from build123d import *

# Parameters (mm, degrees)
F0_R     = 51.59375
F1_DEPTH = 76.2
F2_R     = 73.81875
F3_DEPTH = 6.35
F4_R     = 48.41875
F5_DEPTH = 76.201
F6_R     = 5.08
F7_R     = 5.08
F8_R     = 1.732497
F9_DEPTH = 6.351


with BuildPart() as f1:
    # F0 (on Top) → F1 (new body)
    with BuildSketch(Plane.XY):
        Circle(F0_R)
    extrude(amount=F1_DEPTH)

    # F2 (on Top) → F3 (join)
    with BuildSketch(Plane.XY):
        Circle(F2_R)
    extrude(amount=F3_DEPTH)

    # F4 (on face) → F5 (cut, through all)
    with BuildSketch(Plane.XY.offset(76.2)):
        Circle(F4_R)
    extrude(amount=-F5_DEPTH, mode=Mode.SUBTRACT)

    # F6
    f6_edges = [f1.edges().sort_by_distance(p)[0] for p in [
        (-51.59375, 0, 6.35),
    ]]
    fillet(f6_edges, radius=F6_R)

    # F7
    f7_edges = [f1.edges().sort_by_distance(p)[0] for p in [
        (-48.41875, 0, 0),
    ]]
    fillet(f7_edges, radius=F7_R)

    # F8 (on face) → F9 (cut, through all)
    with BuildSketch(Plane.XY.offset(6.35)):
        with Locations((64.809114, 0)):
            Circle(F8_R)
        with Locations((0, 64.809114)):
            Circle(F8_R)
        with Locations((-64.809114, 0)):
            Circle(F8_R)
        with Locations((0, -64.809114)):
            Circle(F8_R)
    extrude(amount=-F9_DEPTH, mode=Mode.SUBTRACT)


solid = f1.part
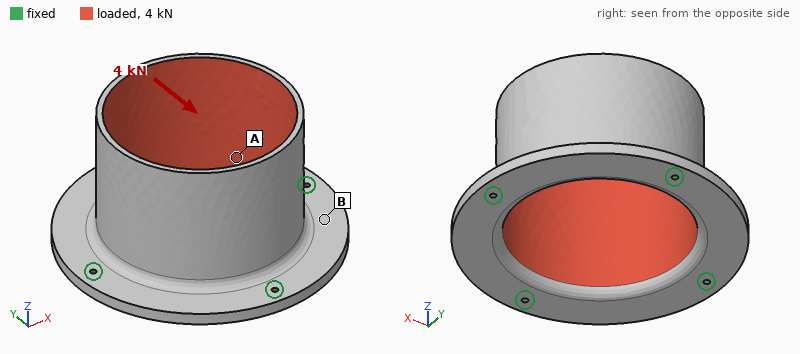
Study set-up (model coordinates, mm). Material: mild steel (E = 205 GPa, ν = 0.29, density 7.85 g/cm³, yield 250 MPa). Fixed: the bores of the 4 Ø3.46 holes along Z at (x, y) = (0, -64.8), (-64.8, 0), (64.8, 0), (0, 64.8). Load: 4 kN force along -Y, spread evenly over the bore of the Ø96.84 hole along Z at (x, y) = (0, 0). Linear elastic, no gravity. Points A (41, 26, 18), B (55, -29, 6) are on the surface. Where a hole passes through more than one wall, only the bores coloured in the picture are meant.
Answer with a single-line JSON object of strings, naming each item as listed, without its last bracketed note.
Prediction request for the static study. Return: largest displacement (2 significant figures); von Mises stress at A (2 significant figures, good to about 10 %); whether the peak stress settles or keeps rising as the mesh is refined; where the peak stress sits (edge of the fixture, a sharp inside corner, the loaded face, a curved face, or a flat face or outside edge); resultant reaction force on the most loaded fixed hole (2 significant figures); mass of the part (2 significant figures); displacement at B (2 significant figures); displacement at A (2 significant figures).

{"largest displacement": "22 µm", "von Mises stress at A": "9.3 MPa", "whether the peak stress settles or keeps rising as the mesh is refined": "keeps rising", "where the peak stress sits": "edge of the fixture", "resultant reaction force on the most loaded fixed hole": "1.5 kN", "mass of the part": "1.0 kg", "displacement at B": "6.4 µm", "displacement at A": "7.7 µm"}
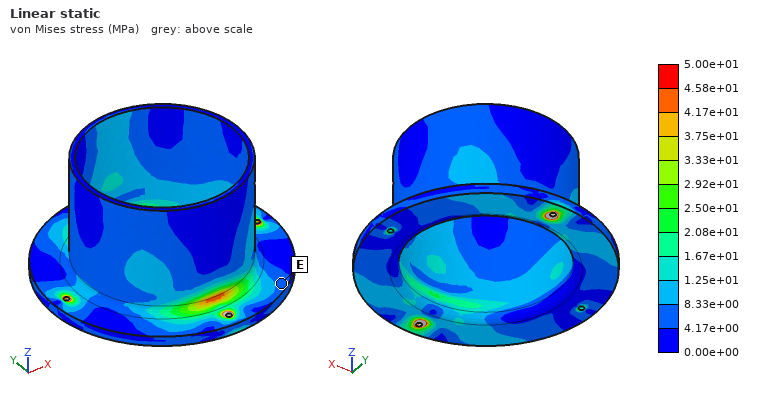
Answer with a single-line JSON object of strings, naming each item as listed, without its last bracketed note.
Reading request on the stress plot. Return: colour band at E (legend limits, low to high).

{"colour band at E": "4.17e+00 to 8.33e+00 MPa"}
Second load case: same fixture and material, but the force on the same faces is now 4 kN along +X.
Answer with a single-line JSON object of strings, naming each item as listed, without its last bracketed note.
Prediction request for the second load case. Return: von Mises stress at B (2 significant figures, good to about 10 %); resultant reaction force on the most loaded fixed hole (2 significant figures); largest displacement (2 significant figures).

{"von Mises stress at B": "12 MPa", "resultant reaction force on the most loaded fixed hole": "1.5 kN", "largest displacement": "22 µm"}
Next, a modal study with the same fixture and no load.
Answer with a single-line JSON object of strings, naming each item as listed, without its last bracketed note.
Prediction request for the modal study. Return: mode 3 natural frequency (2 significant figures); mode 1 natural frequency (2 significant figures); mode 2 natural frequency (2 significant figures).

{"mode 3 natural frequency": "2500 Hz", "mode 1 natural frequency": "1400 Hz", "mode 2 natural frequency": "2500 Hz"}
